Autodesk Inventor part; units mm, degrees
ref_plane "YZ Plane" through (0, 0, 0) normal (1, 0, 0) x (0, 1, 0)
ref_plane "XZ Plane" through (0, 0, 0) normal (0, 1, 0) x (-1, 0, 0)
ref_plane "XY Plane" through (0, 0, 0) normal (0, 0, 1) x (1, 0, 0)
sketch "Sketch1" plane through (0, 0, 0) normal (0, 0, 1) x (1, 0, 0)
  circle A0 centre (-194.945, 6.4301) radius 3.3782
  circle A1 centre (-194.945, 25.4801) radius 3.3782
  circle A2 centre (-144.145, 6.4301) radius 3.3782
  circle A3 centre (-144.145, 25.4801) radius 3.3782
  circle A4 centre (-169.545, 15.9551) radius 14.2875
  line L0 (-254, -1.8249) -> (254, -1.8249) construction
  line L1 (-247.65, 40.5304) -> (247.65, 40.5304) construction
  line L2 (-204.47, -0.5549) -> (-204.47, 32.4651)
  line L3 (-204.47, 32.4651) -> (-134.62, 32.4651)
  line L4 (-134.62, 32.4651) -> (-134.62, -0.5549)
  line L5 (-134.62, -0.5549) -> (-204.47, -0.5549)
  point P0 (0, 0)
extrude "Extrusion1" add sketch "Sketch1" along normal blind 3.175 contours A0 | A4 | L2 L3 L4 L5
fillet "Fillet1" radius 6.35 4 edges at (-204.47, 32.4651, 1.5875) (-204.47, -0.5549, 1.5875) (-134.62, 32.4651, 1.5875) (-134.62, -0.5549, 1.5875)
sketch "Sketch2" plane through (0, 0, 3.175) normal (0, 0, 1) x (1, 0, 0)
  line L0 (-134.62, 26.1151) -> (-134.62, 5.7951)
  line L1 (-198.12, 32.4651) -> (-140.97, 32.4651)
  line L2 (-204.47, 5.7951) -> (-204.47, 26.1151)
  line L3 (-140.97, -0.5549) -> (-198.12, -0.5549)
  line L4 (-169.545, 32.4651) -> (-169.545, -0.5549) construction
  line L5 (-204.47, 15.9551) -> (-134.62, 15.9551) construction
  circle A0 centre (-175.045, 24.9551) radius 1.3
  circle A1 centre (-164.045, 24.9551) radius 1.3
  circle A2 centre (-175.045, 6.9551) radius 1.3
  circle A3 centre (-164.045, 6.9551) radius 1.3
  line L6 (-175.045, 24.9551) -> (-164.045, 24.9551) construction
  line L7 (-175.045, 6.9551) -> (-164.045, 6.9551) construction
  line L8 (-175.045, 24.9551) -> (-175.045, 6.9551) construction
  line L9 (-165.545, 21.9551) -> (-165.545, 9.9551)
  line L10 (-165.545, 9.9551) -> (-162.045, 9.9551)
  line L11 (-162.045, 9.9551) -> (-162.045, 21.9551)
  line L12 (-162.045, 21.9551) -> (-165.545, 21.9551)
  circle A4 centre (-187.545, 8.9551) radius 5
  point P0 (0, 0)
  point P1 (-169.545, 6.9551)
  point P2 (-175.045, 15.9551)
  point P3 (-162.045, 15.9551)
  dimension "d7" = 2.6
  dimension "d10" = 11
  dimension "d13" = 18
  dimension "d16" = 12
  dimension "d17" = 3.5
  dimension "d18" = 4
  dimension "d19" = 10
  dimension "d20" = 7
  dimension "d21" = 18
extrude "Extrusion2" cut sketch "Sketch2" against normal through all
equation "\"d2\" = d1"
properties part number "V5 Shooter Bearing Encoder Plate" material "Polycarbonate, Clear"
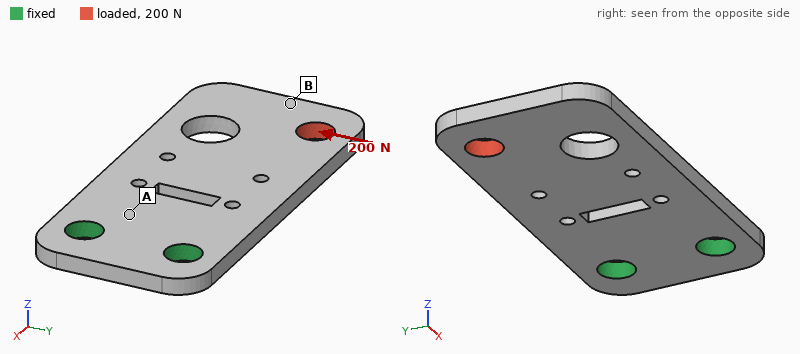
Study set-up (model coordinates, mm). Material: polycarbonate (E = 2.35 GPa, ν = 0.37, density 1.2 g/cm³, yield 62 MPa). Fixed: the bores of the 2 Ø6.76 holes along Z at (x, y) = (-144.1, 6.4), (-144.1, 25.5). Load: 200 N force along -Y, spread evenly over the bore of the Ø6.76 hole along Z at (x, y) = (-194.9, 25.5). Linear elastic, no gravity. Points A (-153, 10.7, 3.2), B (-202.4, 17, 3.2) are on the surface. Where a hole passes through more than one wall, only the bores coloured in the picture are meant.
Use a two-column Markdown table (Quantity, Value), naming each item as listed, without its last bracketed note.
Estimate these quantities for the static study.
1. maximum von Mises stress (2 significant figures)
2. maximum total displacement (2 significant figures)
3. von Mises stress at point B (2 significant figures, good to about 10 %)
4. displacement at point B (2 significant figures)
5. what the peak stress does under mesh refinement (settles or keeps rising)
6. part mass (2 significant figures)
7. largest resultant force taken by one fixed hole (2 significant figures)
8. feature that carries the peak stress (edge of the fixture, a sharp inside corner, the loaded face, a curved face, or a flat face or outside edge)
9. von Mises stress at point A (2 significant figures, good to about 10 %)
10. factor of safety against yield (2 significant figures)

| Quantity | Value |
|---|---|
| maximum von Mises stress | 37 MPa |
| maximum total displacement | 0.75 mm |
| von Mises stress at point B | 2.7 MPa |
| displacement at point B | 0.71 mm |
| what the peak stress does under mesh refinement | settles |
| part mass | 7.7 g |
| largest resultant force taken by one fixed hole | 450 N |
| feature that carries the peak stress | a curved face |
| von Mises stress at point A | 6.9 MPa |
| factor of safety against yield | 1.7 |
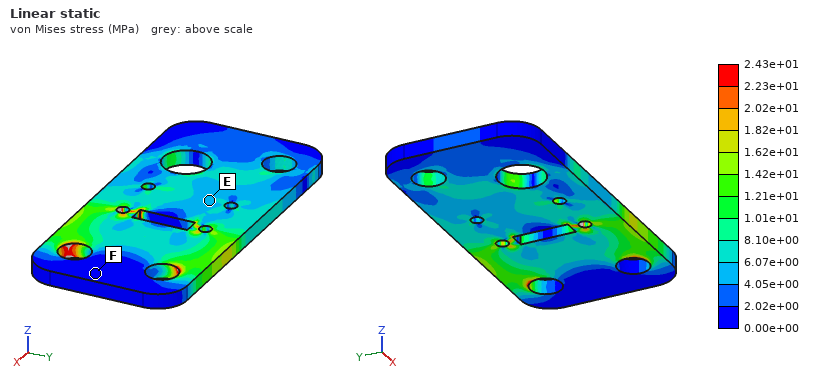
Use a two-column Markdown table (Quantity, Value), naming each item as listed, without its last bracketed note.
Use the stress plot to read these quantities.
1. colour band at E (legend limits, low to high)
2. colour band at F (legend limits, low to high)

| Quantity | Value |
|---|---|
| colour band at E | 4.05e+00 to 6.07e+00 MPa |
| colour band at F | 0.00e+00 to 2.02e+00 MPa |
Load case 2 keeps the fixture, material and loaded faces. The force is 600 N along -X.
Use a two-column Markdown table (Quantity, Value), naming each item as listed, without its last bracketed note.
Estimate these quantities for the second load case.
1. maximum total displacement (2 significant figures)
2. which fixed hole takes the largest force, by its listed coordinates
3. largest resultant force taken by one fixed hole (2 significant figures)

| Quantity | Value |
|---|---|
| maximum total displacement | 0.57 mm |
| which fixed hole takes the largest force, by its listed coordinates | (-144.1, 25.5) |
| largest resultant force taken by one fixed hole | 560 N |
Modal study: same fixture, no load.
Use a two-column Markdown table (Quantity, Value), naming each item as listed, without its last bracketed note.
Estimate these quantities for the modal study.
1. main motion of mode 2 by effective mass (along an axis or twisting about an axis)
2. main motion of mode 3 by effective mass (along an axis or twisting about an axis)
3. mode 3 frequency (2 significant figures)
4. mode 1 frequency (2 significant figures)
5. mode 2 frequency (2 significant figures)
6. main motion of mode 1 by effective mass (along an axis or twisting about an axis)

| Quantity | Value |
|---|---|
| main motion of mode 2 by effective mass | twisting about X |
| main motion of mode 3 by effective mass | along Z |
| mode 3 frequency | 1300 Hz |
| mode 1 frequency | 210 Hz |
| mode 2 frequency | 790 Hz |
| main motion of mode 1 by effective mass | along Z |
